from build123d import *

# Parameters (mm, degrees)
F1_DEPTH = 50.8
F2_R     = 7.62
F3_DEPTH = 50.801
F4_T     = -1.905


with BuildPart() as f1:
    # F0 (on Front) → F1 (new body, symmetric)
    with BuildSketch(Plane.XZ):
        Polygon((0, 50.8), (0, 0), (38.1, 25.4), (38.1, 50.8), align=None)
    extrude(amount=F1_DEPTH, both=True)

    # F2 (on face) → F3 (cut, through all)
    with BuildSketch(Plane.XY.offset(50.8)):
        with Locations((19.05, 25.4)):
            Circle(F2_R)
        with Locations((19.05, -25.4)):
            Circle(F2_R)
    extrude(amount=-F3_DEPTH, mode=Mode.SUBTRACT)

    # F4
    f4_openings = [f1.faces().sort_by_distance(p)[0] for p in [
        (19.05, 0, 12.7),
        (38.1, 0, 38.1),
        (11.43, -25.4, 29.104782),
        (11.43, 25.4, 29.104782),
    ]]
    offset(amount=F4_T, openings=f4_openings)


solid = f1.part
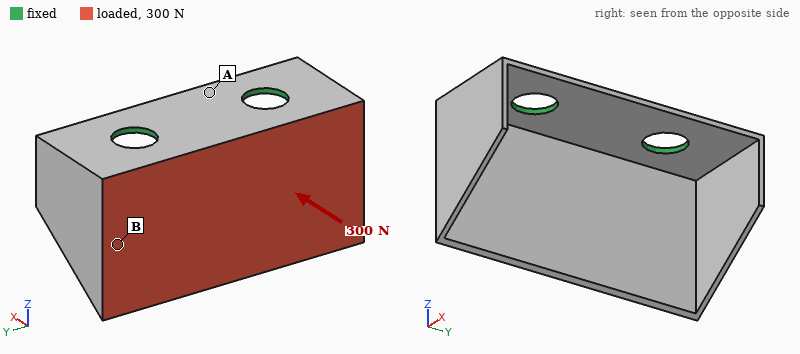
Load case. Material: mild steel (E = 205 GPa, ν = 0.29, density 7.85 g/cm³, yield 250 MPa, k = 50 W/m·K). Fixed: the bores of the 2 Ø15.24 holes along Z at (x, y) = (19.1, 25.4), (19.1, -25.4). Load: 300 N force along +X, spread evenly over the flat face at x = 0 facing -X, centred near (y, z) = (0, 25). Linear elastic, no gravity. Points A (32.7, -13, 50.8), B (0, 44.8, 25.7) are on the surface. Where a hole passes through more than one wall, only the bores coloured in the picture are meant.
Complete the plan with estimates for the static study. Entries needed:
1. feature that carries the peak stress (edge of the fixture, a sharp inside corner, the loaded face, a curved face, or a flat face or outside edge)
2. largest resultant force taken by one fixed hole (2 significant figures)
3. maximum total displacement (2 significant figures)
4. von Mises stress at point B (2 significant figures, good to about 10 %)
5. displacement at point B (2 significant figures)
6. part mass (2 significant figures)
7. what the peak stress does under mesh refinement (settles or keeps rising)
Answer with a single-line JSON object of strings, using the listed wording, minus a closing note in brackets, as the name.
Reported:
{"feature that carries the peak stress": "edge of the fixture", "largest resultant force taken by one fixed hole": "150 N", "maximum total displacement": "0.31 mm", "von Mises stress at point B": "25 MPa", "displacement at point B": "0.087 mm", "part mass": "160 g", "what the peak stress does under mesh refinement": "keeps rising"}
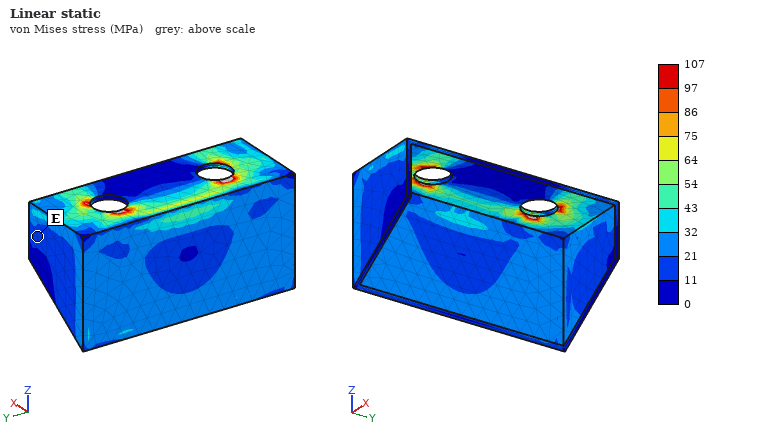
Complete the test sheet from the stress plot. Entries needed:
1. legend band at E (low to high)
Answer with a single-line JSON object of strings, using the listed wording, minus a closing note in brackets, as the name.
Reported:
{"legend band at E": "11 to 21 MPa"}
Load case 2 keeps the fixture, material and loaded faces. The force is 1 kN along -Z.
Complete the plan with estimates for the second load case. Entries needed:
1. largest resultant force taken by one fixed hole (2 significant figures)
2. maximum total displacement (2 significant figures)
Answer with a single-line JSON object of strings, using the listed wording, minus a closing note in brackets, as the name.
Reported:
{"largest resultant force taken by one fixed hole": "500 N", "maximum total displacement": "0.25 mm"}
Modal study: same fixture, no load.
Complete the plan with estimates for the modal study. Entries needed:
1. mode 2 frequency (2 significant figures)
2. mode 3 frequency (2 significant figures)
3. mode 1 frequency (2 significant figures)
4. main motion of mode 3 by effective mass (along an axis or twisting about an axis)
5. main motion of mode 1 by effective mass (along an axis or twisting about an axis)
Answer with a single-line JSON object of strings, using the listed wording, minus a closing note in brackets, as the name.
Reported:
{"mode 2 frequency": "990 Hz", "mode 3 frequency": "1700 Hz", "mode 1 frequency": "700 Hz", "main motion of mode 3 by effective mass": "along Y", "main motion of mode 1 by effective mass": "along X"}
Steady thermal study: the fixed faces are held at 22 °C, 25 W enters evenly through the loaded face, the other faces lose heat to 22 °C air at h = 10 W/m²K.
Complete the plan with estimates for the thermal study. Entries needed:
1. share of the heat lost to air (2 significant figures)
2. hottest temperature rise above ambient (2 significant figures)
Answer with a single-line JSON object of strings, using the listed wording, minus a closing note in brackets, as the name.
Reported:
{"share of the heat lost to air": "22 %", "hottest temperature rise above ambient": "71 K"}
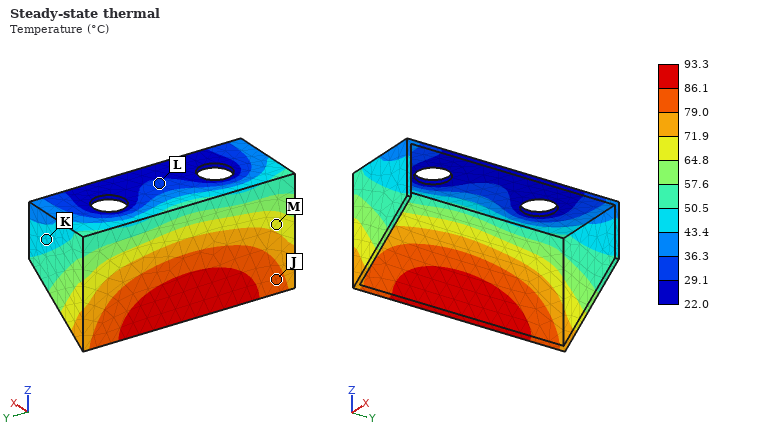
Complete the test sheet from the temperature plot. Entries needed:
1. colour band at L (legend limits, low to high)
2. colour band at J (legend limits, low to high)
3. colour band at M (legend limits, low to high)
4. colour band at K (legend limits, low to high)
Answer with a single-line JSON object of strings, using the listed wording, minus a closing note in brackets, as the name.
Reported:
{"colour band at L": "29.1 to 36.3 °C", "colour band at J": "79.0 to 86.1 °C", "colour band at M": "64.8 to 71.9 °C", "colour band at K": "43.4 to 50.5 °C"}
